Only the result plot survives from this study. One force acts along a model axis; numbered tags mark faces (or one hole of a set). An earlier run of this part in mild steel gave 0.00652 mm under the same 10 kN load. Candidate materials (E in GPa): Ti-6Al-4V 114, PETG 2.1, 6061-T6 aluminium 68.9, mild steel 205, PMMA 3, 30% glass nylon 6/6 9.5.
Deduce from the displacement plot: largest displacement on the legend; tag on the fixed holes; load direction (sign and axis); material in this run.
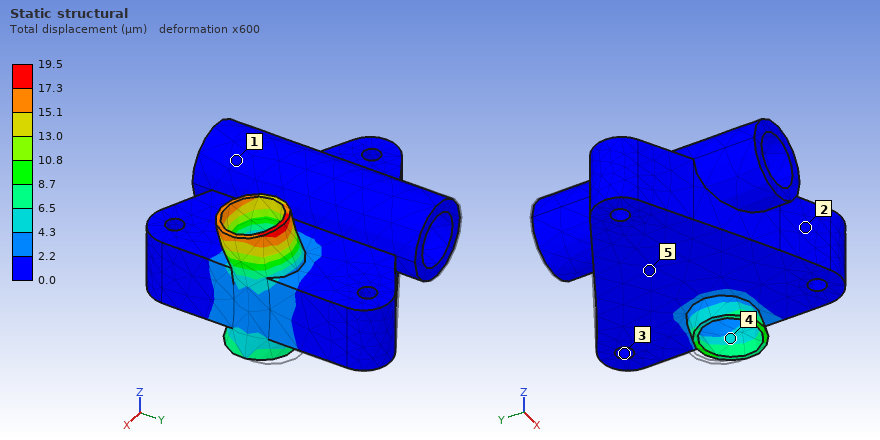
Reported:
19.5 µm
3
-Y
6061-T6 aluminium
